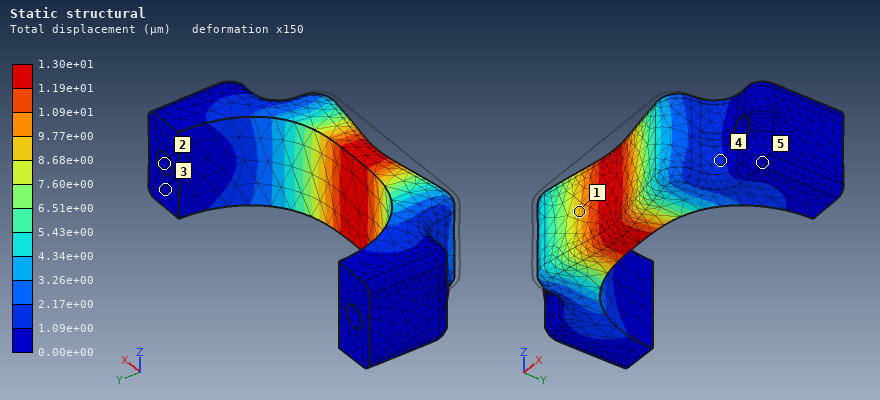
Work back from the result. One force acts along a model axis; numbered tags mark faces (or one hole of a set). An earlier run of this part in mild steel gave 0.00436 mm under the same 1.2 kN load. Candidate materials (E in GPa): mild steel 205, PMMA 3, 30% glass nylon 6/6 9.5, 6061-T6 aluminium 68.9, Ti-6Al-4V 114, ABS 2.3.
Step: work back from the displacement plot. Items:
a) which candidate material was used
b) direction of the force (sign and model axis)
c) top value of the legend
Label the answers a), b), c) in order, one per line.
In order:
a) 6061-T6 aluminium
b) +Y
c) 1.30e+01 µm
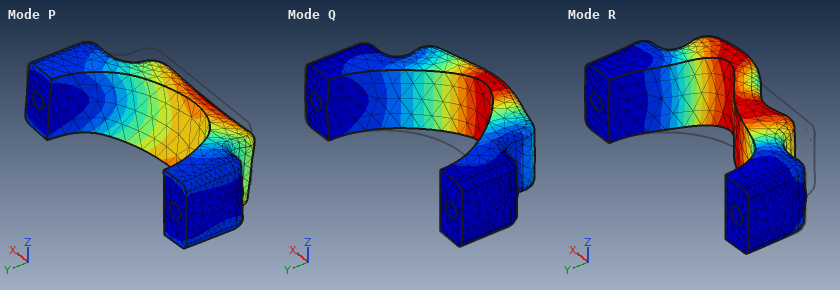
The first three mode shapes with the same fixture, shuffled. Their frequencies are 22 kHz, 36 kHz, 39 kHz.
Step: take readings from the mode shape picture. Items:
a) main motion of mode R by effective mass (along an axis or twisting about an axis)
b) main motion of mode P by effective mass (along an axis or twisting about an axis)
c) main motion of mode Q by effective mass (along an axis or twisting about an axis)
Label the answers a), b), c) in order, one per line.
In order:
a) along X
b) along Z
c) along Y
